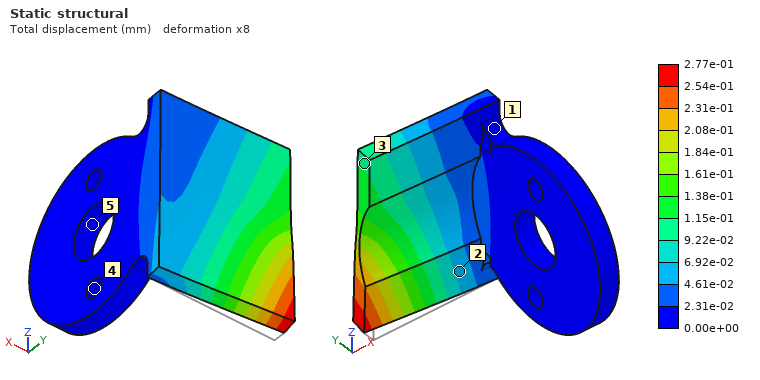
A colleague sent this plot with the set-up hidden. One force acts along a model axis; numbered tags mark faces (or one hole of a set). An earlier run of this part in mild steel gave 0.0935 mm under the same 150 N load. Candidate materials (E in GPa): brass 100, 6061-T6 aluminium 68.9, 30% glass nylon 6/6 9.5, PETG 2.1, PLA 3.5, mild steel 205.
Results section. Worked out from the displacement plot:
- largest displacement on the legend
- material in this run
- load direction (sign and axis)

2.77e-01 mm
6061-T6 aluminium
+Y
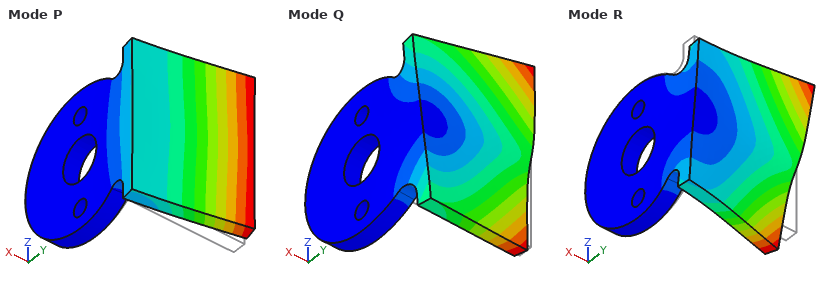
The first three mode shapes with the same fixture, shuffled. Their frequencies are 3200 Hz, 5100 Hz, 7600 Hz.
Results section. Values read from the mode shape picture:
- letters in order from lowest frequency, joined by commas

P, Q, R
